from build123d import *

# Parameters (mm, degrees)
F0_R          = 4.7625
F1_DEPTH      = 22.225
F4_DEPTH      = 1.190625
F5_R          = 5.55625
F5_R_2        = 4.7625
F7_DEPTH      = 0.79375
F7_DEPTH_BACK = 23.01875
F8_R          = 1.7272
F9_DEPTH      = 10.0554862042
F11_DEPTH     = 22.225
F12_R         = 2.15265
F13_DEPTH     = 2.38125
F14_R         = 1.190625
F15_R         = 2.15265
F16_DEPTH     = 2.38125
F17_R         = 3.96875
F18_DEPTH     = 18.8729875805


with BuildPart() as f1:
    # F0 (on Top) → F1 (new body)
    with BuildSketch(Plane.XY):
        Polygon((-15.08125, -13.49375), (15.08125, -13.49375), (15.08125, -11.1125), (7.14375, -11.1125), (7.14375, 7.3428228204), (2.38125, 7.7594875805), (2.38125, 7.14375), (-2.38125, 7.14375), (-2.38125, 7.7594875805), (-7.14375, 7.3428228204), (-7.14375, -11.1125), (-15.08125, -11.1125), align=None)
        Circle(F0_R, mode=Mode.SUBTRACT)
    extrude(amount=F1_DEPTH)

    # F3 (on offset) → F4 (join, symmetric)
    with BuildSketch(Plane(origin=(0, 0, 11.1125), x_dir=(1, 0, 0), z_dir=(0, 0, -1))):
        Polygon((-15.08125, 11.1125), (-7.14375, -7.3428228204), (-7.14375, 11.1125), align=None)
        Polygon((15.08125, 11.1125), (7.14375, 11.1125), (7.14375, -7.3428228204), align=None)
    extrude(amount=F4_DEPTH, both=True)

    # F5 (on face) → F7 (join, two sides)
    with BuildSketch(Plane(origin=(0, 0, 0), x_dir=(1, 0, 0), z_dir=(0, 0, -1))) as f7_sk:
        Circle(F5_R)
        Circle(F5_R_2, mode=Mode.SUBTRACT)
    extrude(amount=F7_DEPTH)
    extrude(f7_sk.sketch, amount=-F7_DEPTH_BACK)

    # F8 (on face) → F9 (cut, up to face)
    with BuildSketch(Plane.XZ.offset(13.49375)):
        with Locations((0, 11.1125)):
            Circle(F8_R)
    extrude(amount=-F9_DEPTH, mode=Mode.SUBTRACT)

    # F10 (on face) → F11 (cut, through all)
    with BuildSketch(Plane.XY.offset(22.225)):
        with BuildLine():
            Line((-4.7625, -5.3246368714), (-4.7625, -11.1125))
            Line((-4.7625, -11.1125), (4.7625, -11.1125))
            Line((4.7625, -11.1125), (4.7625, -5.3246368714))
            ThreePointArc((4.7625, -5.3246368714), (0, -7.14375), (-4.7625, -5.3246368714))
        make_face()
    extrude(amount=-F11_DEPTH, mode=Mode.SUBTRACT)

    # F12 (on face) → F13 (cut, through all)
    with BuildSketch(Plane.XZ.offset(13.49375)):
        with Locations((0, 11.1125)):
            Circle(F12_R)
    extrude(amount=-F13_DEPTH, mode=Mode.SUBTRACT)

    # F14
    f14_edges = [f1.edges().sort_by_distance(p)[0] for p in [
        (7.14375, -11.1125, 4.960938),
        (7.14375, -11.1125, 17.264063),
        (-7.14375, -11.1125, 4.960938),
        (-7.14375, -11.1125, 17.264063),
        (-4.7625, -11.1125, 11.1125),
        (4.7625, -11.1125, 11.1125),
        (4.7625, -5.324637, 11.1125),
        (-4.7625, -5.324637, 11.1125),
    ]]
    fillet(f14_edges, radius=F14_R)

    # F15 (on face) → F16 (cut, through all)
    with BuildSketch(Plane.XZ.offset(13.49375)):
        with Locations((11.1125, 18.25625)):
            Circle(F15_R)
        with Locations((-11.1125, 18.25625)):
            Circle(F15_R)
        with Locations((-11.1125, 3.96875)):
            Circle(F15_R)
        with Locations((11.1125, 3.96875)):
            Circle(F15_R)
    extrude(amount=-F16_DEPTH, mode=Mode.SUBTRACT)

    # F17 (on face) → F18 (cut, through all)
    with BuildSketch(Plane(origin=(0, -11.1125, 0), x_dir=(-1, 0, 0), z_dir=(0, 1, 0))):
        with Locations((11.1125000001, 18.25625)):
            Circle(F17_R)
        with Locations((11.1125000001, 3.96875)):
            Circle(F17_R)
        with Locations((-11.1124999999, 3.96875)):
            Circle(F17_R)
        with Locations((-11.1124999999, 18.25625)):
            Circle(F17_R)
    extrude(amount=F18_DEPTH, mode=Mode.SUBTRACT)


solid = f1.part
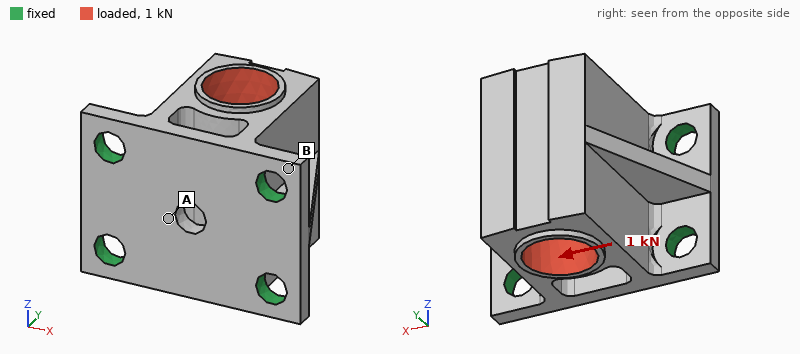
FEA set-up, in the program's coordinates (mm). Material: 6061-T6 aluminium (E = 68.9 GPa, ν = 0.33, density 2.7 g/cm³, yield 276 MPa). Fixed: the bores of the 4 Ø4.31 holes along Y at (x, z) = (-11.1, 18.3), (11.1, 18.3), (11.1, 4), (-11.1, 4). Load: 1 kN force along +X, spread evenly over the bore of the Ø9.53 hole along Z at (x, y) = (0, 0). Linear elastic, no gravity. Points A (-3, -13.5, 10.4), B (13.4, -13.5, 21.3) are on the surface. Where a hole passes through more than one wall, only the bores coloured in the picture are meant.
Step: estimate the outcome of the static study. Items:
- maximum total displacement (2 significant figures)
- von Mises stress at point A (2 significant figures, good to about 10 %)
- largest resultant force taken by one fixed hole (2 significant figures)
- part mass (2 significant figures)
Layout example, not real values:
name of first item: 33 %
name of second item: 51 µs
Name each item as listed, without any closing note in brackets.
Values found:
maximum total displacement: 19 µm
von Mises stress at point A: 8.5 MPa
largest resultant force taken by one fixed hole: 390 N
part mass: 14 g
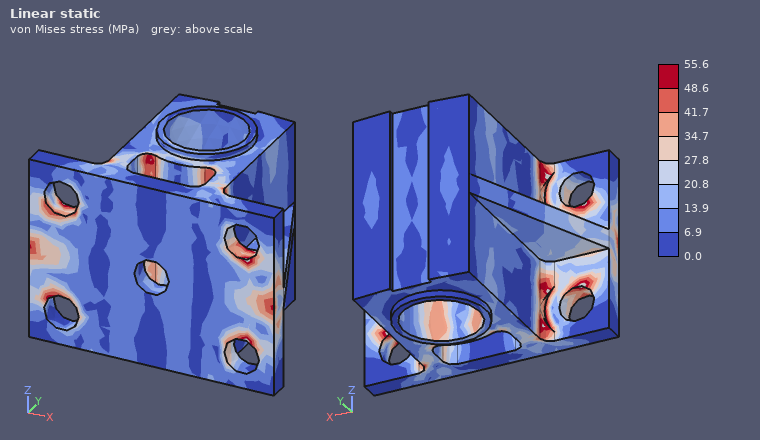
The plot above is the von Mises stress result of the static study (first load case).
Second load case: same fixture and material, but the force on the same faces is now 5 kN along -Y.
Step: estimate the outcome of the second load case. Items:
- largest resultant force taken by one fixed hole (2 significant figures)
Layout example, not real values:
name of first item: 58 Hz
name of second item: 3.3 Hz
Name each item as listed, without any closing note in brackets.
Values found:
largest resultant force taken by one fixed hole: 1.3 kN
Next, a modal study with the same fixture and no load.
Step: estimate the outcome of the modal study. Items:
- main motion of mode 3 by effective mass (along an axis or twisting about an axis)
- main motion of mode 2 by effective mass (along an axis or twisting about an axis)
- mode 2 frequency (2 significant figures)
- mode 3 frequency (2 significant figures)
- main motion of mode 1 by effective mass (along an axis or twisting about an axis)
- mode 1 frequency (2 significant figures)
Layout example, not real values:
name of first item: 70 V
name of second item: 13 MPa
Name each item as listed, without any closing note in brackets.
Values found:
main motion of mode 3 by effective mass: twisting about Y
main motion of mode 2 by effective mass: along X
mode 2 frequency: 14 kHz
mode 3 frequency: 19 kHz
main motion of mode 1 by effective mass: along Z
mode 1 frequency: 12 kHz
